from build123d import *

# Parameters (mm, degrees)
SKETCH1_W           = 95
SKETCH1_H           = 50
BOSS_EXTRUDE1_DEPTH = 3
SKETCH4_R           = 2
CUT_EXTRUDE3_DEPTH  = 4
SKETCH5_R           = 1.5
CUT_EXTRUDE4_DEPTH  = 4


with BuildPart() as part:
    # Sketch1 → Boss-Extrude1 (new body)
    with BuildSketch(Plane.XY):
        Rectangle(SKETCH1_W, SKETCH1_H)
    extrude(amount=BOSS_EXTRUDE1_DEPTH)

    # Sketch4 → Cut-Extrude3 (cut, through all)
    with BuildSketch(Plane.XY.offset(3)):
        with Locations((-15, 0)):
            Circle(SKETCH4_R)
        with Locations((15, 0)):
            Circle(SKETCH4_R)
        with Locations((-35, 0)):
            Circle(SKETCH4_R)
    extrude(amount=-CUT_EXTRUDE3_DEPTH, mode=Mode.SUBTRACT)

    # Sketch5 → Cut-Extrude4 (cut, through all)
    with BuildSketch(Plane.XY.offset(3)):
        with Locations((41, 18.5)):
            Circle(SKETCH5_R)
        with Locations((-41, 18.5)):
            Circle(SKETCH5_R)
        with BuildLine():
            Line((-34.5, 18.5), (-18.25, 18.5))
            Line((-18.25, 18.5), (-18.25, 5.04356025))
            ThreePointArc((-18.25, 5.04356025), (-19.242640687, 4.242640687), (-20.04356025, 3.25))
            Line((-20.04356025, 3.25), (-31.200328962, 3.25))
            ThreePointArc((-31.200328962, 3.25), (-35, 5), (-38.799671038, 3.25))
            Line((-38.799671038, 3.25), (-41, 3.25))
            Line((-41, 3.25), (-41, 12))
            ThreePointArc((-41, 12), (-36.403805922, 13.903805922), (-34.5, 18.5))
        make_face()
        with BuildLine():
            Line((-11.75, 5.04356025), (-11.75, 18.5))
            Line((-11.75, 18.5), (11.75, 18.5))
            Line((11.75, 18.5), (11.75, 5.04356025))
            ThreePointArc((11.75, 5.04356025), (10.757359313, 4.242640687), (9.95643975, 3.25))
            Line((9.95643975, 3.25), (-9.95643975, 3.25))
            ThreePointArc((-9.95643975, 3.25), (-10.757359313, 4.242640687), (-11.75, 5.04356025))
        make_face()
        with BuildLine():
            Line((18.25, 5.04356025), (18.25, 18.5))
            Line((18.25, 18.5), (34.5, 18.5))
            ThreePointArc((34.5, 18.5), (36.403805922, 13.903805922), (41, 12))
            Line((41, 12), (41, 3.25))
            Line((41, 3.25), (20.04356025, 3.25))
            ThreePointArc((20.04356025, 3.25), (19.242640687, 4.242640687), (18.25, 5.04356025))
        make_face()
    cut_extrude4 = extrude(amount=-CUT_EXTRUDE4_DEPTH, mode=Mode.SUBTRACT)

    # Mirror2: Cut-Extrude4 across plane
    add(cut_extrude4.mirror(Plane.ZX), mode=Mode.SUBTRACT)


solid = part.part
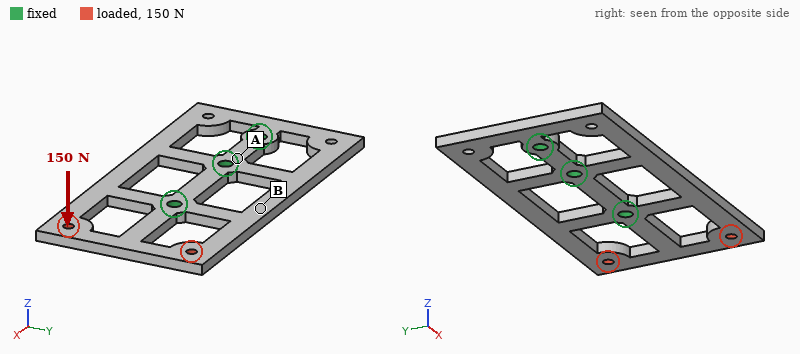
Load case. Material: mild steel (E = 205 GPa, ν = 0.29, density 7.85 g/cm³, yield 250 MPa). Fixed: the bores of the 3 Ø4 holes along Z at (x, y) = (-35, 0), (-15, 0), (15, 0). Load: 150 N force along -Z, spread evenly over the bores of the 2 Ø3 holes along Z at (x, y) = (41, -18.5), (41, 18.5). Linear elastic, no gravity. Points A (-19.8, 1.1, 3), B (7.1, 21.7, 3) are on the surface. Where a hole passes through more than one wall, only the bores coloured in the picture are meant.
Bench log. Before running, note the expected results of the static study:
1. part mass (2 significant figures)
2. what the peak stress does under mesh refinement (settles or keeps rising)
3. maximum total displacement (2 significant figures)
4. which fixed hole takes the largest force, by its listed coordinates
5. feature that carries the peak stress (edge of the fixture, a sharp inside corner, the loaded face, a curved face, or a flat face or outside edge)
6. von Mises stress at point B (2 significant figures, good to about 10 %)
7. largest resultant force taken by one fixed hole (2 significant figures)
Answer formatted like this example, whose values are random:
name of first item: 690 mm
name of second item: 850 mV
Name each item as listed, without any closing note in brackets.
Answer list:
part mass: 65 g
what the peak stress does under mesh refinement: keeps rising
maximum total displacement: 0.20 mm
which fixed hole takes the largest force, by its listed coordinates: (15, 0)
feature that carries the peak stress: edge of the fixture
von Mises stress at point B: 40 MPa
largest resultant force taken by one fixed hole: 180 N
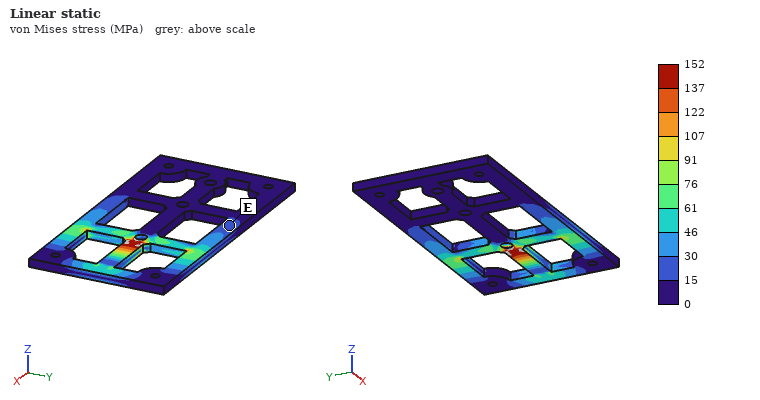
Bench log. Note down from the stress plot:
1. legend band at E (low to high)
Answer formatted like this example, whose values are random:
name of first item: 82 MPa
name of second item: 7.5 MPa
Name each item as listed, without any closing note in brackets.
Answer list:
legend band at E: 15 to 30 MPa
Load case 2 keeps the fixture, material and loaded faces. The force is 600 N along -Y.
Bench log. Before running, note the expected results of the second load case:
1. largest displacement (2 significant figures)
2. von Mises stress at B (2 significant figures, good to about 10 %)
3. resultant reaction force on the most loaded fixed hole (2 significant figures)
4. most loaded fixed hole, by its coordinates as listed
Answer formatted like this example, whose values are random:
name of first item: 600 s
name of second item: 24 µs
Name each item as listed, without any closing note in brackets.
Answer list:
largest displacement: 40 µm
von Mises stress at B: 15 MPa
resultant reaction force on the most loaded fixed hole: 810 N
most loaded fixed hole, by its coordinates as listed: (15, 0)
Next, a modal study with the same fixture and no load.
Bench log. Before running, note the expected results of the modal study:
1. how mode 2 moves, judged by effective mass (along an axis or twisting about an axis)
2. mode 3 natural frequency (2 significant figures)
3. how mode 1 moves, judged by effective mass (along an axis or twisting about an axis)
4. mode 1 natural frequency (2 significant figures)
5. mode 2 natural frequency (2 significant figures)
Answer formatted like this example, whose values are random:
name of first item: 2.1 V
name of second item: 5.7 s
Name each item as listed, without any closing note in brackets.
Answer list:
how mode 2 moves, judged by effective mass: twisting about X
mode 3 natural frequency: 2300 Hz
how mode 1 moves, judged by effective mass: along Z
mode 1 natural frequency: 1400 Hz
mode 2 natural frequency: 1800 Hz
